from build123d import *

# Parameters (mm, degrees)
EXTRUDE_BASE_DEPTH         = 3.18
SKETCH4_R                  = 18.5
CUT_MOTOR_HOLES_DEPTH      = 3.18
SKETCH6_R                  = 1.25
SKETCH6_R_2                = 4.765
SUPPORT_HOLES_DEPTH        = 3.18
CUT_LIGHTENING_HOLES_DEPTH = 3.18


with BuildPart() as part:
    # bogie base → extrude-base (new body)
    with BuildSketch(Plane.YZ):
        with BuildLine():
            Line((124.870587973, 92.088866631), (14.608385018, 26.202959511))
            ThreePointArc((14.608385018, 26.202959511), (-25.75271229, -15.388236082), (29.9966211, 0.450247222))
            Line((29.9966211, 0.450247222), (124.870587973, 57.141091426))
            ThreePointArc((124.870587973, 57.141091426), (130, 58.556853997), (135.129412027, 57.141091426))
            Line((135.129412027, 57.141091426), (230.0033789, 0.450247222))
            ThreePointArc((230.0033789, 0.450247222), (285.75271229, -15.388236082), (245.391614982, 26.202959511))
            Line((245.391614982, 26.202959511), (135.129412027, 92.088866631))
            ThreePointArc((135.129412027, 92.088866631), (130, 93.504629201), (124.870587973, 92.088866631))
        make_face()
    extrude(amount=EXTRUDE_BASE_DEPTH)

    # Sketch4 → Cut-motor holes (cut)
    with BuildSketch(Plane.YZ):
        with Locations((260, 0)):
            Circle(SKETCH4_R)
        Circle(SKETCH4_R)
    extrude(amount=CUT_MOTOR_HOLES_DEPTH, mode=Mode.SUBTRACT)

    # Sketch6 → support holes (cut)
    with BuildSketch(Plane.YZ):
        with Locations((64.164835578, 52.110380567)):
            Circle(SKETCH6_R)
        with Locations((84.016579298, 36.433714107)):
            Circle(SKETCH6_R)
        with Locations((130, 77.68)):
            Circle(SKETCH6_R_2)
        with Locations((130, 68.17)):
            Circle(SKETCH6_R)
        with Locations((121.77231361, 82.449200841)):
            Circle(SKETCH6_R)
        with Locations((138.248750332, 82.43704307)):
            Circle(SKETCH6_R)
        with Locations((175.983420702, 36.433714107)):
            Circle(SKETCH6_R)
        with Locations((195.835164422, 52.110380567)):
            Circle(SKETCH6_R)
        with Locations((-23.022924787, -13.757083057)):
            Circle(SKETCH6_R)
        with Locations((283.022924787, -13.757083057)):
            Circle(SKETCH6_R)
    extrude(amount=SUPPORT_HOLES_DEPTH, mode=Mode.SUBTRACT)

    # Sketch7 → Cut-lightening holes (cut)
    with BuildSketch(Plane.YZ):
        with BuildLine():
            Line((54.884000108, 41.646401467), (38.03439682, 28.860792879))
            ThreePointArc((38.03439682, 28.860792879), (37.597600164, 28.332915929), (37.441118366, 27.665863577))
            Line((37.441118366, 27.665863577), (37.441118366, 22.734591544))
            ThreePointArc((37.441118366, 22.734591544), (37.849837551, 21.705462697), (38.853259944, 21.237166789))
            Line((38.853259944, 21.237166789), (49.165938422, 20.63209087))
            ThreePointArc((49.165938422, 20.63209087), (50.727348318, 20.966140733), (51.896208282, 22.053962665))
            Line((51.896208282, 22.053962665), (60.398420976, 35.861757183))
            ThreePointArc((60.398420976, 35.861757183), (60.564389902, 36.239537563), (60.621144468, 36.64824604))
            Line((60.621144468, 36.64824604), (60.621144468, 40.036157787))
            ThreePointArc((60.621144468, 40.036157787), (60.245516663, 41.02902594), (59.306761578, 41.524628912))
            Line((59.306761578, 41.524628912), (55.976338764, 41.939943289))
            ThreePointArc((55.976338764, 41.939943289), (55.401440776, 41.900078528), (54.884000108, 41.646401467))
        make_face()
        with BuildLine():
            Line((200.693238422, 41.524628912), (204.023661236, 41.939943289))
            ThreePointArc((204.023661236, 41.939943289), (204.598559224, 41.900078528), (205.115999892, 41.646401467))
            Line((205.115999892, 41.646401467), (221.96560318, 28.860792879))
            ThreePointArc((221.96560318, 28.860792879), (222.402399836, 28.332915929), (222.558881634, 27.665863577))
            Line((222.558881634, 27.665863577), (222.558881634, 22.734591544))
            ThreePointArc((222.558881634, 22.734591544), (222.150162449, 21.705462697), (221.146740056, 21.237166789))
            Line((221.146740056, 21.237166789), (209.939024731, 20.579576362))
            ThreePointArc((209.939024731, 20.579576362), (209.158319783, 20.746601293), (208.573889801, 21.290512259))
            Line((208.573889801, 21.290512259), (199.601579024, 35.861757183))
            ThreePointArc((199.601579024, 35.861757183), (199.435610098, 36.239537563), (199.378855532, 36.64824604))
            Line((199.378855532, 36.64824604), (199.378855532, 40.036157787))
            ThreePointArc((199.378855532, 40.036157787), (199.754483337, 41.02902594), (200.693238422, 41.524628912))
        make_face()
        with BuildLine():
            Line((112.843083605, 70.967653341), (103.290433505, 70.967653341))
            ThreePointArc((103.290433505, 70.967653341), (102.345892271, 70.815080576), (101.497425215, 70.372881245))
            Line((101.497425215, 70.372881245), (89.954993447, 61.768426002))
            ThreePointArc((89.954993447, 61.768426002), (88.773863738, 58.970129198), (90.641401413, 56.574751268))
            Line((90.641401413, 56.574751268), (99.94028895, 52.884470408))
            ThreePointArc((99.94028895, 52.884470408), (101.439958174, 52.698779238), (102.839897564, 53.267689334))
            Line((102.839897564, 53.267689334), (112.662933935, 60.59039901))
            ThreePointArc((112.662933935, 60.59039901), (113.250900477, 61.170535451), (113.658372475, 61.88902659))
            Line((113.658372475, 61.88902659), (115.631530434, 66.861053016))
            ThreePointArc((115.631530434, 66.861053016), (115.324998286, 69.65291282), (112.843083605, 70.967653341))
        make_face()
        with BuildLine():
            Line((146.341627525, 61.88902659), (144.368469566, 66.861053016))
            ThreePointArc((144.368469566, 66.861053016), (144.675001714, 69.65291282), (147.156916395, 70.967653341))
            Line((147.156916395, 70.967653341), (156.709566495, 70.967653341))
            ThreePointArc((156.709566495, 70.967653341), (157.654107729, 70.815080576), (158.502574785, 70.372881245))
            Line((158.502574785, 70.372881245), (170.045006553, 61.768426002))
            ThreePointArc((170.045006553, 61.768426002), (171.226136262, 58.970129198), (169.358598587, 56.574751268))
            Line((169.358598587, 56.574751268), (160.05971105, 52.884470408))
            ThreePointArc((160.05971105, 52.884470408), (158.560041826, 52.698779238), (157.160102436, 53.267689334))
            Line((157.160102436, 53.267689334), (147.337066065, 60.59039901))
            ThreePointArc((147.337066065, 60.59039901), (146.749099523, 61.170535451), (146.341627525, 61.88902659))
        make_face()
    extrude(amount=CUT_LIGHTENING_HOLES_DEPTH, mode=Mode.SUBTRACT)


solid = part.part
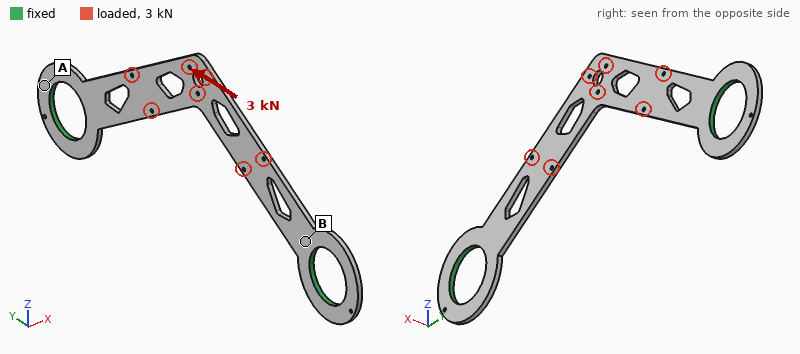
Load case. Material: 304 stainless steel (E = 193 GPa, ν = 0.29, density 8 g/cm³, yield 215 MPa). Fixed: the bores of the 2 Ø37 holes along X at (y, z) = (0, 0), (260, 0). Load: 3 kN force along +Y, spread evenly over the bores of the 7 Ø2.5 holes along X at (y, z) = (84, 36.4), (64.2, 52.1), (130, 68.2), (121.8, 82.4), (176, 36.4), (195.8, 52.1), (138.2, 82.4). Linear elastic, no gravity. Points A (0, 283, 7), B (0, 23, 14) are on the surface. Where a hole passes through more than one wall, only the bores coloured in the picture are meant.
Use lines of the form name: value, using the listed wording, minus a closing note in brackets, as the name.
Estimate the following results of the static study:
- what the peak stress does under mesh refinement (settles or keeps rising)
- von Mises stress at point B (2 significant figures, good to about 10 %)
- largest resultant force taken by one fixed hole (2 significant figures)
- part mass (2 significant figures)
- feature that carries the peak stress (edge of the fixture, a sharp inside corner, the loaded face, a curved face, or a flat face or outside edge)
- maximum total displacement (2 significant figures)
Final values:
what the peak stress does under mesh refinement: keeps rising
von Mises stress at point B: 16 MPa
largest resultant force taken by one fixed hole: 1.6 kN
part mass: 240 g
feature that carries the peak stress: a sharp inside corner
maximum total displacement: 24 µm
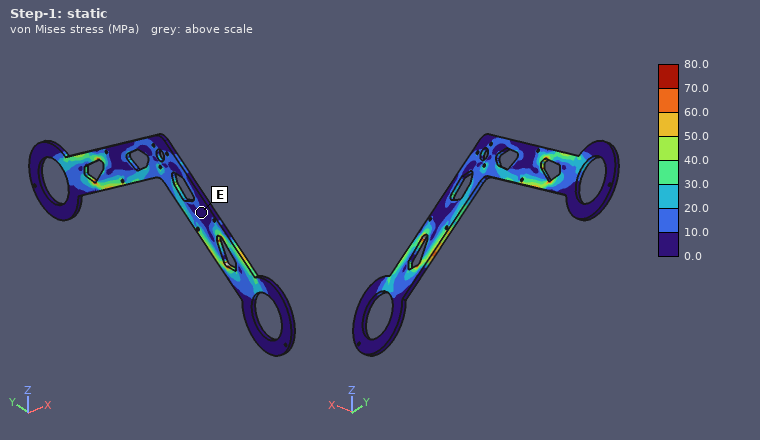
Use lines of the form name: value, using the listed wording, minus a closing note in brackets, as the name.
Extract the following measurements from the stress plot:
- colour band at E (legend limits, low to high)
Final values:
colour band at E: 0.0 to 10.0 MPa
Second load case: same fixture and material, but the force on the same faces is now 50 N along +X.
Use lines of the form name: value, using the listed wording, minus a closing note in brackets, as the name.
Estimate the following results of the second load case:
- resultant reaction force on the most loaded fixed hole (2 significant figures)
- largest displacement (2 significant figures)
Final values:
resultant reaction force on the most loaded fixed hole: 25 N
largest displacement: 0.47 mm
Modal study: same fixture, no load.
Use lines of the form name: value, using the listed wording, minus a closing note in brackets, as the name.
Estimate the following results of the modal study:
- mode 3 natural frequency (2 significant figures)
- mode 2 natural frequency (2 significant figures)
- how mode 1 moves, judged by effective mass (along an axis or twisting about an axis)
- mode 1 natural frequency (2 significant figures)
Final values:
mode 3 natural frequency: 910 Hz
mode 2 natural frequency: 640 Hz
how mode 1 moves, judged by effective mass: along X
mode 1 natural frequency: 200 Hz
